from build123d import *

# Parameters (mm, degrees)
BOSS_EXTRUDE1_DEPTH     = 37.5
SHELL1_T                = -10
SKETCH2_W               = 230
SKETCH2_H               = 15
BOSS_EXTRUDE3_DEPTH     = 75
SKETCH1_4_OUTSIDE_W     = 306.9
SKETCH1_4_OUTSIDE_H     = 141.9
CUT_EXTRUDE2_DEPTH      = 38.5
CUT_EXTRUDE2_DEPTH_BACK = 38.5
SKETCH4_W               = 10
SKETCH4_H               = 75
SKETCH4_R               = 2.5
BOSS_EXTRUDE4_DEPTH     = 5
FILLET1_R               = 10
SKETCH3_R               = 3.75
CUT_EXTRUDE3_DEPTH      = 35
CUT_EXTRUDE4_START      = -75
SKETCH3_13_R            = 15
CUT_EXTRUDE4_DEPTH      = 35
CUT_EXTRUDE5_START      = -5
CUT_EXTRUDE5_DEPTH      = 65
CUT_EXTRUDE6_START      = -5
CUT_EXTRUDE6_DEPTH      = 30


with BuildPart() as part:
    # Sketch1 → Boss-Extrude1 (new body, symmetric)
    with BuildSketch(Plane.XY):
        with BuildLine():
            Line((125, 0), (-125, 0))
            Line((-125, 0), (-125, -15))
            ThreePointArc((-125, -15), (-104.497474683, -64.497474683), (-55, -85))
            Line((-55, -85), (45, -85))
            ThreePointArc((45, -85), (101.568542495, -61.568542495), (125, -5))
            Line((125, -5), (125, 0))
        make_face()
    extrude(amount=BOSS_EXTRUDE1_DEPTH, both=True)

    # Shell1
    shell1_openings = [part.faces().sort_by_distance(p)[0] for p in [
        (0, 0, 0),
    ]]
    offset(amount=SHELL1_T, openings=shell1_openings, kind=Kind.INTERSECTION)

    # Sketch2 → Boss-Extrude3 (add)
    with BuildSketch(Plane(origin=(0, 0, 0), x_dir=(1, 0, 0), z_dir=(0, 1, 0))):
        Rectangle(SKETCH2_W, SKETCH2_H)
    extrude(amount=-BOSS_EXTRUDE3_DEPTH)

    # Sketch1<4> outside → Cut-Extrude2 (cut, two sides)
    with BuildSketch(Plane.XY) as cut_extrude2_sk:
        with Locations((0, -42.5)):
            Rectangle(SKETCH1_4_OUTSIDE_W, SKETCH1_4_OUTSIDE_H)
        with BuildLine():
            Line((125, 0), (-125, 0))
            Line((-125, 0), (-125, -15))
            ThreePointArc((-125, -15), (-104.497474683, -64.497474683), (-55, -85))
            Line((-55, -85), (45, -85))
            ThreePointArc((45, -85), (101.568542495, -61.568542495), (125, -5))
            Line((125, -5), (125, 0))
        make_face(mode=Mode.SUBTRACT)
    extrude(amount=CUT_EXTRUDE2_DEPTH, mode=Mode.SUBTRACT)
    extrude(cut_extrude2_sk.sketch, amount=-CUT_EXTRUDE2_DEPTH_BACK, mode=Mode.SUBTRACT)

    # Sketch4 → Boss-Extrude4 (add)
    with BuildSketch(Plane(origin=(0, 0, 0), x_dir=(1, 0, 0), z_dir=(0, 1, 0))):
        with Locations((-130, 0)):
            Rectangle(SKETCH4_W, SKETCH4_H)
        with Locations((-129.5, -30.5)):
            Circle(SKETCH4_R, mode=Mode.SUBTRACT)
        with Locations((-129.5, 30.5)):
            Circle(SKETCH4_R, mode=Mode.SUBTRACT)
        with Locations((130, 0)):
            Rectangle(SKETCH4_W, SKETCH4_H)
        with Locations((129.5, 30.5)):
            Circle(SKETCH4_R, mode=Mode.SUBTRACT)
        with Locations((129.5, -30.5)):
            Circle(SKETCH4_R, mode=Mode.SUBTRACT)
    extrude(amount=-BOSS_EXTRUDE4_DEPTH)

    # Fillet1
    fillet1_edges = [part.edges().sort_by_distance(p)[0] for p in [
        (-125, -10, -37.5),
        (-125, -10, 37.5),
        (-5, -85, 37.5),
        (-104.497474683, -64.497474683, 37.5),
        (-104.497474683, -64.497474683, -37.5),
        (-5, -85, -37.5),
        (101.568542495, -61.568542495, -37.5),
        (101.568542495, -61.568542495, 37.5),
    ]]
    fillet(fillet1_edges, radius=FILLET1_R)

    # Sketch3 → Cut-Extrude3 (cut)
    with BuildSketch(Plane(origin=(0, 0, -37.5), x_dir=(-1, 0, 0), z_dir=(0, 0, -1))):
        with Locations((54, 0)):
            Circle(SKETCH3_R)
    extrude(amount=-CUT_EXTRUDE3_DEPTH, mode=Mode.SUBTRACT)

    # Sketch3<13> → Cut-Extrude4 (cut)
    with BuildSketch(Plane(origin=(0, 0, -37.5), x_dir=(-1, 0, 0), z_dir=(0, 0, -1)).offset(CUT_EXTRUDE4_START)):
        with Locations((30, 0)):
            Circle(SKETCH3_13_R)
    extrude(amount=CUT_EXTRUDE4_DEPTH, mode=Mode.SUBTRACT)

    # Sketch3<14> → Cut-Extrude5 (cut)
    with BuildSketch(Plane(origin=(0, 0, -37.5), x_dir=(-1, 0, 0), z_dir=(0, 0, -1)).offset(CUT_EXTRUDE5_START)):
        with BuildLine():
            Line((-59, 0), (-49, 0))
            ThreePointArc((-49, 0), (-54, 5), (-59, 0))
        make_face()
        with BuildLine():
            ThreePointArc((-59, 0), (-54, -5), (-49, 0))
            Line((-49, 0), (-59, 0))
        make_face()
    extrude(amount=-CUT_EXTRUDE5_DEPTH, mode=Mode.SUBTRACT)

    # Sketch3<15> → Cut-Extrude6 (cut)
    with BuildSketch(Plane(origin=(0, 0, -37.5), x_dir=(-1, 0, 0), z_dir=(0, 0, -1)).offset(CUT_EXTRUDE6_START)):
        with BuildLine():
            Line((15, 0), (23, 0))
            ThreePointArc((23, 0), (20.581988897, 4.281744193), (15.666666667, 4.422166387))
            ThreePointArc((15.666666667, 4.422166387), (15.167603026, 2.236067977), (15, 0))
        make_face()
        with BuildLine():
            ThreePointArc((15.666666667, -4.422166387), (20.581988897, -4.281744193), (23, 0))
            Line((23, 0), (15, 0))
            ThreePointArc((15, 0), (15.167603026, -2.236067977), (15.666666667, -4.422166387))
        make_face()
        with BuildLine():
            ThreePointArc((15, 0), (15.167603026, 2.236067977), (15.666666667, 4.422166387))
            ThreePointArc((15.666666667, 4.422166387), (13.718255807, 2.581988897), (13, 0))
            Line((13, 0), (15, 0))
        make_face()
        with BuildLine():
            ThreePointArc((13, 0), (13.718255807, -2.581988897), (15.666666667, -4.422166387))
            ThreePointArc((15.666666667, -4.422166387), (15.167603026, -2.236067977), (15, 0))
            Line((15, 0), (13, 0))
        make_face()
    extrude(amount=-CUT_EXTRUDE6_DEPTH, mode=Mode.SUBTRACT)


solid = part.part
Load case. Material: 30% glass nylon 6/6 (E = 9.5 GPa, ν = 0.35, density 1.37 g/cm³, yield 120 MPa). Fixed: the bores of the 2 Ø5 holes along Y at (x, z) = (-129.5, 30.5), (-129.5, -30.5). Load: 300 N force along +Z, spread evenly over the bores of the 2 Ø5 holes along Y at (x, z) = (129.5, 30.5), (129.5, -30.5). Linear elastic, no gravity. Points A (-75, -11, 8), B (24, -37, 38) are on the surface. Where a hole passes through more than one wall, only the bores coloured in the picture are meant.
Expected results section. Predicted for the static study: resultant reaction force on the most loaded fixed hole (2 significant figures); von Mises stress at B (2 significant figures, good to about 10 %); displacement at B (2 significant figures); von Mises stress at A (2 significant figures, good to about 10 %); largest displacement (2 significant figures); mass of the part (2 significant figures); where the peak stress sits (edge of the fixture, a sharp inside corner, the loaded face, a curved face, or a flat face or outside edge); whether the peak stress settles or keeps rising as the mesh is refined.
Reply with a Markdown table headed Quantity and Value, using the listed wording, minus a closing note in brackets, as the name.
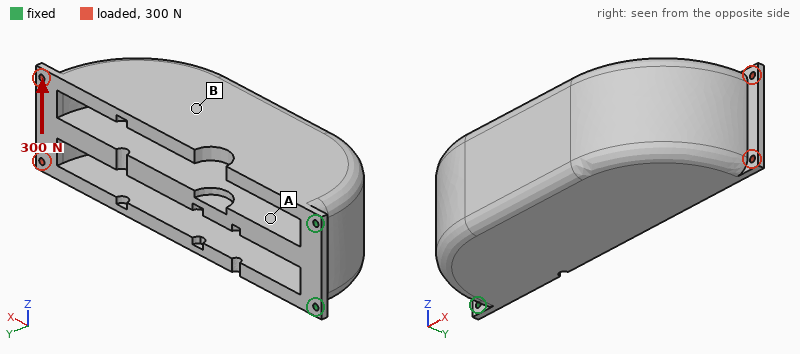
| Quantity | Value |
|---|---|
| resultant reaction force on the most loaded fixed hole | 1.3 kN |
| von Mises stress at B | 2.7 MPa |
| displacement at B | 0.94 mm |
| von Mises stress at A | 5.5 MPa |
| largest displacement | 1.9 mm |
| mass of the part | 1.1 kg |
| where the peak stress sits | edge of the fixture |
| whether the peak stress settles or keeps rising as the mesh is refined | keeps rising |
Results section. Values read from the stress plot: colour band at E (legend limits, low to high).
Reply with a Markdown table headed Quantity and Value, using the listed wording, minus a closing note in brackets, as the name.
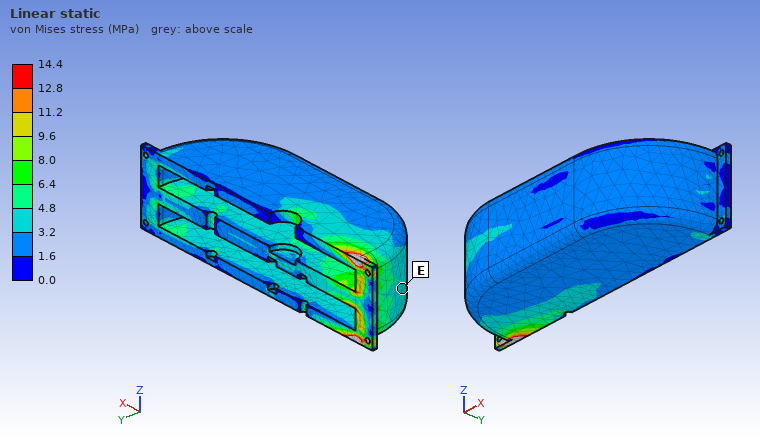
| Quantity | Value |
|---|---|
| colour band at E | 3.2 to 4.8 MPa |
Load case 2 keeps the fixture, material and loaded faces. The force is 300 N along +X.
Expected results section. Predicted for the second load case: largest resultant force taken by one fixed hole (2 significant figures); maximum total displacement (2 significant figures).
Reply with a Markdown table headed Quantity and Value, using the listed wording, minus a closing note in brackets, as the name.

| Quantity | Value |
|---|---|
| largest resultant force taken by one fixed hole | 150 N |
| maximum total displacement | 90 µm |
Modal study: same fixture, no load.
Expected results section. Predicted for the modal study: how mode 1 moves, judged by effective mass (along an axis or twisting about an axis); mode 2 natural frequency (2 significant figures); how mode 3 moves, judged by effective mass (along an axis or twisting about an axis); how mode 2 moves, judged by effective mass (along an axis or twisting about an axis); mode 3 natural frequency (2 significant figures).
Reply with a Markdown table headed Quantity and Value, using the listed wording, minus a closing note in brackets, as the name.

| Quantity | Value |
|---|---|
| how mode 1 moves, judged by effective mass | along Y |
| mode 2 natural frequency | 130 Hz |
| how mode 3 moves, judged by effective mass | along Z |
| how mode 2 moves, judged by effective mass | along Z |
| mode 3 natural frequency | 500 Hz |
